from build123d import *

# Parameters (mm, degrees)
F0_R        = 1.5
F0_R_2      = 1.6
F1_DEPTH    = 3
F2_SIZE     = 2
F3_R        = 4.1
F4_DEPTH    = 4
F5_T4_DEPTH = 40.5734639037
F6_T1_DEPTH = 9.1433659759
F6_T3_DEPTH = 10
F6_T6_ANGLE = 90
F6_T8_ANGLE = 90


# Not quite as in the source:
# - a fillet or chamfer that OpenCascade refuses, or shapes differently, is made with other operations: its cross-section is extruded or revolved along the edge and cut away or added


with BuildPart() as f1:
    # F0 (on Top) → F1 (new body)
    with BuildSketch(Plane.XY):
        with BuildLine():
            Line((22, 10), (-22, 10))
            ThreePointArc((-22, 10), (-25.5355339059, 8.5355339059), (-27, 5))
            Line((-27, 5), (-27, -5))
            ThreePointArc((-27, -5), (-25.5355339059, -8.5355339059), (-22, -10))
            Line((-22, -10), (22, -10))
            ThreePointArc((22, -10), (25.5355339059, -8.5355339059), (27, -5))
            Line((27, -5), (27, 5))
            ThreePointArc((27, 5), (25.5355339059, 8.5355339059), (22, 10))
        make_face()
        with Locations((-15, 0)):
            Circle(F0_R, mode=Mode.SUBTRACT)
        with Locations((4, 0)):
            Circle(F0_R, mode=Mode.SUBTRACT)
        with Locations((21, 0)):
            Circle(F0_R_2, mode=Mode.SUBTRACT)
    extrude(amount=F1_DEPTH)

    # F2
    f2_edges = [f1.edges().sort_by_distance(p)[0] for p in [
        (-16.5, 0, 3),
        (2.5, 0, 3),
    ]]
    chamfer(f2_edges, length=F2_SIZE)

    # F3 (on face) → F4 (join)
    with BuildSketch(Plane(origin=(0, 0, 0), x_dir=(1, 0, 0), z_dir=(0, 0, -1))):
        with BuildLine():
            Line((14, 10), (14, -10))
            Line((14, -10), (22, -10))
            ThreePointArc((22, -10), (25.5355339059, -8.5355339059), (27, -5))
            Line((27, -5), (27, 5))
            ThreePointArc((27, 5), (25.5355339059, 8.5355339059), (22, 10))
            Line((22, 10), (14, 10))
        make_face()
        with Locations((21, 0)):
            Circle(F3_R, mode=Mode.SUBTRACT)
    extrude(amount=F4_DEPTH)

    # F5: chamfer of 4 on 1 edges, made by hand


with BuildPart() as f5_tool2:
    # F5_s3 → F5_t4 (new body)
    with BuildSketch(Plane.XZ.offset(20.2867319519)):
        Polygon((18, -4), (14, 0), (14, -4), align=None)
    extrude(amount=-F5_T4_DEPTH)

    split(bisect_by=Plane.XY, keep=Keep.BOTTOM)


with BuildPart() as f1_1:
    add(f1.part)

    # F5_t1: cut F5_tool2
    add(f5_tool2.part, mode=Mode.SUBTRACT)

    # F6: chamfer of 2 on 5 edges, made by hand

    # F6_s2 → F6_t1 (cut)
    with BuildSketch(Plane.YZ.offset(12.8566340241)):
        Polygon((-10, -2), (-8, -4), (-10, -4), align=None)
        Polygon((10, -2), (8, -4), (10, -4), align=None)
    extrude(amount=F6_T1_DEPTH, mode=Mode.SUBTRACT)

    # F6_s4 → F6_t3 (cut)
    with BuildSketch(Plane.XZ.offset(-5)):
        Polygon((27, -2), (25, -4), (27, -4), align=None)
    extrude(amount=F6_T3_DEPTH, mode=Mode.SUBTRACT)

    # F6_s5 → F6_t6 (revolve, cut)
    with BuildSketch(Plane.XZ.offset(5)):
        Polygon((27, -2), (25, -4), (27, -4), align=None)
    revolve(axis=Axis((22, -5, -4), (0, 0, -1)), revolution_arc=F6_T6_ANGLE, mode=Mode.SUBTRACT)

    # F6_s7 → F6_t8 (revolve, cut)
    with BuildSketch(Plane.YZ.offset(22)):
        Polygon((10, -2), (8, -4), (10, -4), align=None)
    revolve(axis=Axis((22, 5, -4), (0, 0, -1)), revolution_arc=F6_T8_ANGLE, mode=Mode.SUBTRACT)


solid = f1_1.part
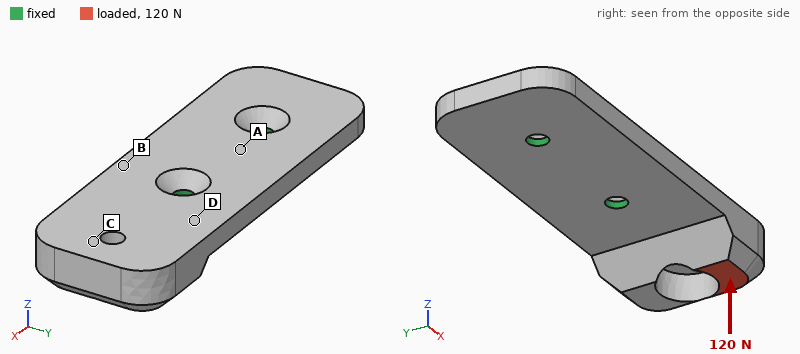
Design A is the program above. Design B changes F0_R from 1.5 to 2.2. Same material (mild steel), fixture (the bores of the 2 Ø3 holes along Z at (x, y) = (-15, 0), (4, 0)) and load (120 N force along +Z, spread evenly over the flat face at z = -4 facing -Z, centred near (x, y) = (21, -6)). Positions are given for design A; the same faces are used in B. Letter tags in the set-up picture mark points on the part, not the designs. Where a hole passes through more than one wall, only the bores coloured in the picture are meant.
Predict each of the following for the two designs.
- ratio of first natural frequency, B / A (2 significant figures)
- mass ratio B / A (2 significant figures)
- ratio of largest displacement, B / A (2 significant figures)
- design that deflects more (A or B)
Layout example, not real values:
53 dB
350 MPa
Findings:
1.1
0.98
0.90
A
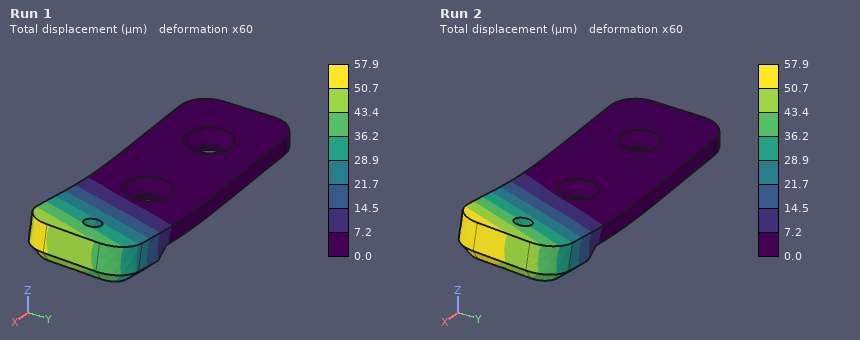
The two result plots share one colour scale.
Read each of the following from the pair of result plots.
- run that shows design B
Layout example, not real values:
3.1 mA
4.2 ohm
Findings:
Run 1
